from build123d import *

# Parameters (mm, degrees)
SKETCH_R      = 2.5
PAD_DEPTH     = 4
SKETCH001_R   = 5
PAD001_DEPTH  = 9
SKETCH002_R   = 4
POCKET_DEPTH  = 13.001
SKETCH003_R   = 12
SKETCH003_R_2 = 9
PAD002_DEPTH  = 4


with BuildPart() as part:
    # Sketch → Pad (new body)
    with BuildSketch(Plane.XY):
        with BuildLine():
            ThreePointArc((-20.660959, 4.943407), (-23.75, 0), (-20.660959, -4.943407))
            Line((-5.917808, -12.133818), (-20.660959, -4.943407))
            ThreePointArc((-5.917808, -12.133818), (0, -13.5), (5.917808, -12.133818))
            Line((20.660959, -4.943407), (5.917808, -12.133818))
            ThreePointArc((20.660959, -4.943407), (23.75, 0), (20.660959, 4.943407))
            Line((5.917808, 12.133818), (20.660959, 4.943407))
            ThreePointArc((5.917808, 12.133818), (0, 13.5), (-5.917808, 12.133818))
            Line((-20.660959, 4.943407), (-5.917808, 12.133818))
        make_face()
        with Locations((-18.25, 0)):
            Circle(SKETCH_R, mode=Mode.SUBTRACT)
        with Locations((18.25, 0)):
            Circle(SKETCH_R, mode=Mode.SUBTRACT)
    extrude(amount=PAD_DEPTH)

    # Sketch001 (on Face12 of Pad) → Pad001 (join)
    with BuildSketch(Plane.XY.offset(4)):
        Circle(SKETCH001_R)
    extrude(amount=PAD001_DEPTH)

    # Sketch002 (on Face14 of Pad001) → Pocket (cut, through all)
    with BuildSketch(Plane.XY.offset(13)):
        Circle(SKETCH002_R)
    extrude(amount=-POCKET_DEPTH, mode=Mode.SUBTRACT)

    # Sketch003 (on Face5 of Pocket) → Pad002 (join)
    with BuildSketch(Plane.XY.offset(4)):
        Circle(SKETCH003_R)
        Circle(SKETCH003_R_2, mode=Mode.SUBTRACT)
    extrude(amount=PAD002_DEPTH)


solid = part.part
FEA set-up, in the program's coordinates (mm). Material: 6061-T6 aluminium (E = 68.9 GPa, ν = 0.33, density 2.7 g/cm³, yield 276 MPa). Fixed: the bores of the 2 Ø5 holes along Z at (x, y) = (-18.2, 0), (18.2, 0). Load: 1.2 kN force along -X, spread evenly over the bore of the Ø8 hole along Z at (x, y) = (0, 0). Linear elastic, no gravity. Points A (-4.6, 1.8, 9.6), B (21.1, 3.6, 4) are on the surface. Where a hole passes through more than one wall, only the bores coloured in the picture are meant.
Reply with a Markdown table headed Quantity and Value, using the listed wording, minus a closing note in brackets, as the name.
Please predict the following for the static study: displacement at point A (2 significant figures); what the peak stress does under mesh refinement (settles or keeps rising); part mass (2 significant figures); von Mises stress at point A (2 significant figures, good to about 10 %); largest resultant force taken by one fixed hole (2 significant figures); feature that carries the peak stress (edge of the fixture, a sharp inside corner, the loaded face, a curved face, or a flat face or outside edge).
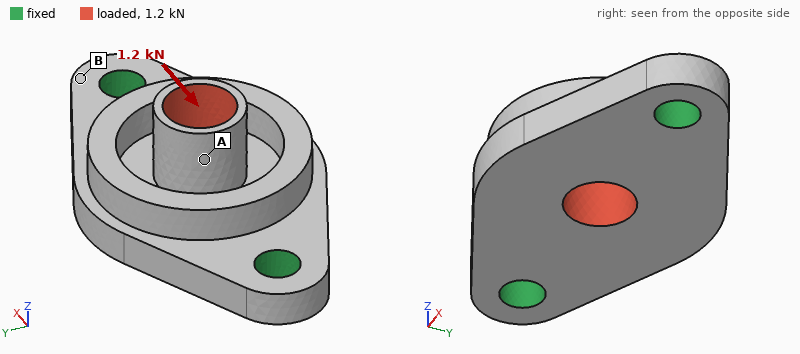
| Quantity | Value |
|---|---|
| displacement at point A | 24 µm |
| what the peak stress does under mesh refinement | keeps rising |
| part mass | 11 g |
| von Mises stress at point A | 22 MPa |
| largest resultant force taken by one fixed hole | 630 N |
| feature that carries the peak stress | a sharp inside corner |
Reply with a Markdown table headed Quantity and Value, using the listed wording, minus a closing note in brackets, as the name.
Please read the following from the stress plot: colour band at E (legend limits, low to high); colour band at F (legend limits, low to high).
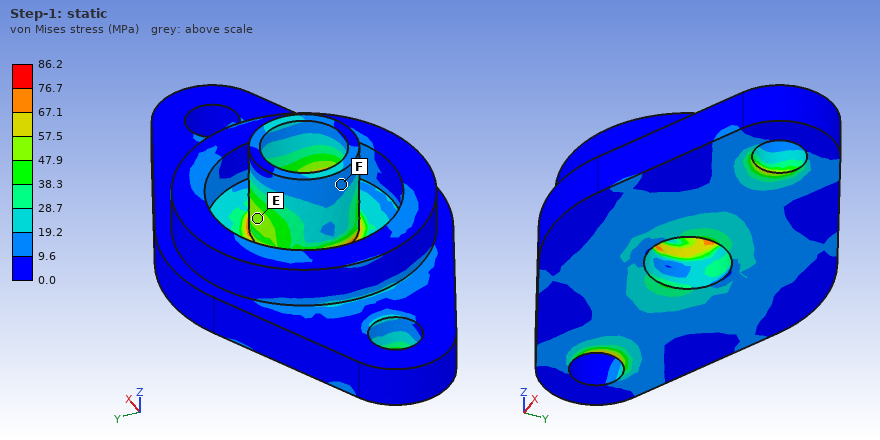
| Quantity | Value |
|---|---|
| colour band at E | 47.9 to 57.5 MPa |
| colour band at F | 9.6 to 19.2 MPa |
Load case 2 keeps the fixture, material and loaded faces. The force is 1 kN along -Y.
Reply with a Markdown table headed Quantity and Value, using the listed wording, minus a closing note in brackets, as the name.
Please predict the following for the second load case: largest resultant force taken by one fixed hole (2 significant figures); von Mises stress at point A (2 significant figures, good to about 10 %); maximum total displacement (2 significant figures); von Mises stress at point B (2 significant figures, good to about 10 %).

| Quantity | Value |
|---|---|
| largest resultant force taken by one fixed hole | 500 N |
| von Mises stress at point A | 29 MPa |
| maximum total displacement | 51 µm |
| von Mises stress at point B | 9.4 MPa |
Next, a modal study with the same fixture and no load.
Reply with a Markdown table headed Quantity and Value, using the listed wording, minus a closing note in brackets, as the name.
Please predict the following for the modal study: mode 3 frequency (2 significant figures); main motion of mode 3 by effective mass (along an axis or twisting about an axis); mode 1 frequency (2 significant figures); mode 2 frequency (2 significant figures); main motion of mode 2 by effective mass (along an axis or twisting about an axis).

| Quantity | Value |
|---|---|
| mode 3 frequency | 28 kHz |
| main motion of mode 3 by effective mass | along Y |
| mode 1 frequency | 11 kHz |
| mode 2 frequency | 13 kHz |
| main motion of mode 2 by effective mass | along Z |
